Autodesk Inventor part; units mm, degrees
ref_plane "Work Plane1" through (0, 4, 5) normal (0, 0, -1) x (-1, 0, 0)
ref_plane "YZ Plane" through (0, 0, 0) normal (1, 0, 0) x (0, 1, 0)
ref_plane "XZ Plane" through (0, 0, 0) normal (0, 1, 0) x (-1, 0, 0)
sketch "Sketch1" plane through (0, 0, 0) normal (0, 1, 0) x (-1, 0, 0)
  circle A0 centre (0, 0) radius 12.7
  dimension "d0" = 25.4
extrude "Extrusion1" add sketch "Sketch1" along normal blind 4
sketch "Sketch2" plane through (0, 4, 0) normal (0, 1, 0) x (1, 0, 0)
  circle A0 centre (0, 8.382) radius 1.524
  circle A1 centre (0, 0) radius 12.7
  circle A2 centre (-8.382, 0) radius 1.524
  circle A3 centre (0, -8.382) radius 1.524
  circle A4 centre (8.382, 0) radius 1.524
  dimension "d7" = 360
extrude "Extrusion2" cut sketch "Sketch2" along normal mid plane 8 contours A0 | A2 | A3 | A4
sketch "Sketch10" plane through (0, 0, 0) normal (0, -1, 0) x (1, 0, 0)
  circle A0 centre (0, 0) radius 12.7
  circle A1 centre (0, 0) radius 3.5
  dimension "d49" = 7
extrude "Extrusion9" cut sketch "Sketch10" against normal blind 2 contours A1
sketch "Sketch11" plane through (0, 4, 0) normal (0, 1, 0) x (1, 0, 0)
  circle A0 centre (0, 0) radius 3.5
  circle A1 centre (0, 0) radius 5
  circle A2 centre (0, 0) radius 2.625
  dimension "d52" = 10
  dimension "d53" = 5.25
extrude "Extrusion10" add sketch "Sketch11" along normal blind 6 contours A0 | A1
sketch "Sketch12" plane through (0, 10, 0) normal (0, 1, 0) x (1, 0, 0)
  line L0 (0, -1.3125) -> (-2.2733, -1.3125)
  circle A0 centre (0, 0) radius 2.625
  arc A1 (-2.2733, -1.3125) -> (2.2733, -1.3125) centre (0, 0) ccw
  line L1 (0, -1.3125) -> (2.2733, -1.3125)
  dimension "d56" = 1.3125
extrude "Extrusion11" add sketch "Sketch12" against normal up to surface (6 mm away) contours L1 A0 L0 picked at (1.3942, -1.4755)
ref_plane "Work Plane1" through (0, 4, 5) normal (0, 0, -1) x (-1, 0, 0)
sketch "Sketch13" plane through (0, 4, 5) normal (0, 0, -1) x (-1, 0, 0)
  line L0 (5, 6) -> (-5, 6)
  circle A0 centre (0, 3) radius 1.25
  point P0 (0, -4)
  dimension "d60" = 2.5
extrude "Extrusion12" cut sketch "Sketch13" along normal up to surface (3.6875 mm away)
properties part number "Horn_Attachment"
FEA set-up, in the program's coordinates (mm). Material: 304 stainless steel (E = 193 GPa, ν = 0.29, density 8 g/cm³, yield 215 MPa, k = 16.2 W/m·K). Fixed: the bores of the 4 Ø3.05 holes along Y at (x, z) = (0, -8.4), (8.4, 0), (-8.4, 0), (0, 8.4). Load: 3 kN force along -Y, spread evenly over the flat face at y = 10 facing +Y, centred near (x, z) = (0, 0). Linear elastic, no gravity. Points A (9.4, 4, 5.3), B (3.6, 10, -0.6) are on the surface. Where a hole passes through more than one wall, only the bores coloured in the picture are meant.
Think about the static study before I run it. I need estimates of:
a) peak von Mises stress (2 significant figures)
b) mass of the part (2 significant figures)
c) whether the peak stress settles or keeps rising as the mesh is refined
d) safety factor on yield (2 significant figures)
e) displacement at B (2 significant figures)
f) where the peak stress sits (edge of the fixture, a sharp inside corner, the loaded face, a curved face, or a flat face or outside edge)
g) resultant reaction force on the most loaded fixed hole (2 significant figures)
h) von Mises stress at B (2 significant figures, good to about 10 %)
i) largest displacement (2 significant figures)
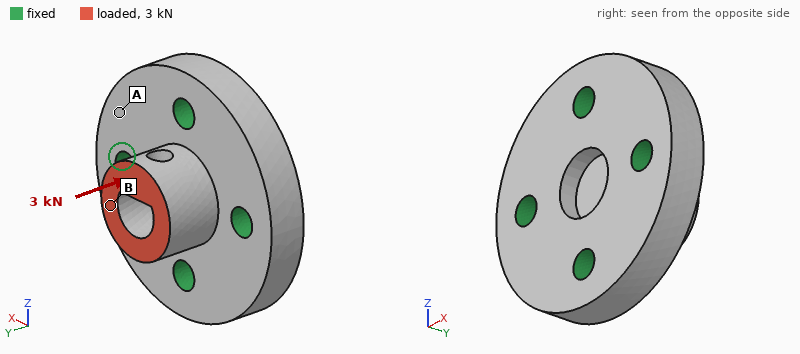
210 MPa
17 g
settles
1.0
3.6 µm
a curved face
820 N
53 MPa
5.3 µm
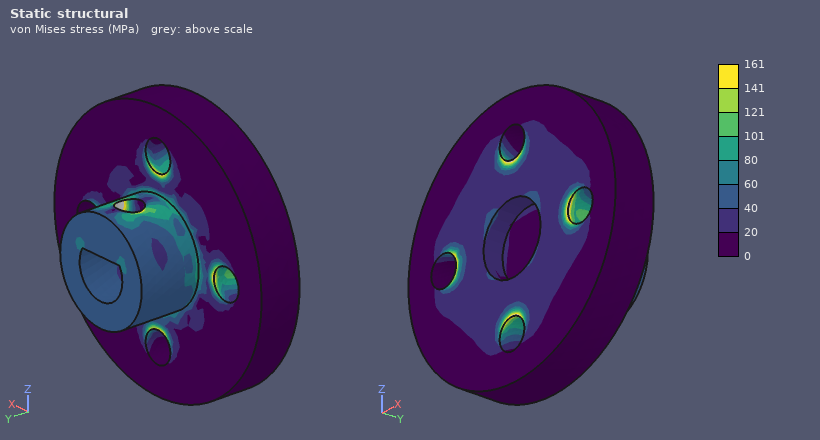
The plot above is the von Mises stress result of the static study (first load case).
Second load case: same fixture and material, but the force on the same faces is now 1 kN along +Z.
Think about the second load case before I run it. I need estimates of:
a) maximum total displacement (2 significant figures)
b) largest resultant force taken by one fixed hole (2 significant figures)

7.5 µm
630 N
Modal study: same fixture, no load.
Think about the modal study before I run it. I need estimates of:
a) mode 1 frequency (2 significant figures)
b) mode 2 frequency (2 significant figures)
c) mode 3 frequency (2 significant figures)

60 kHz
60 kHz
65 kHz
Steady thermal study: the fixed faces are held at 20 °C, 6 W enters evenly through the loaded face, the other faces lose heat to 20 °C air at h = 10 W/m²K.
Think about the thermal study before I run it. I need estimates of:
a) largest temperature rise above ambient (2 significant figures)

61 K
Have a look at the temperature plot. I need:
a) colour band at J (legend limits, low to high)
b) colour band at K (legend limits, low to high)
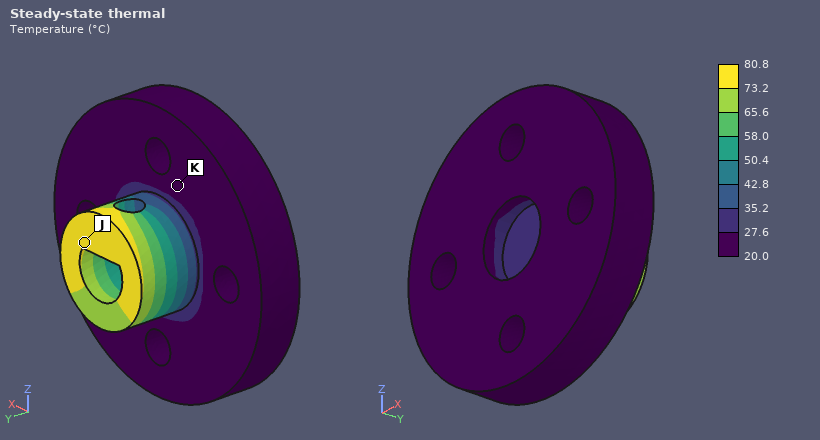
73.2 to 80.8 °C
20.0 to 27.6 °C
